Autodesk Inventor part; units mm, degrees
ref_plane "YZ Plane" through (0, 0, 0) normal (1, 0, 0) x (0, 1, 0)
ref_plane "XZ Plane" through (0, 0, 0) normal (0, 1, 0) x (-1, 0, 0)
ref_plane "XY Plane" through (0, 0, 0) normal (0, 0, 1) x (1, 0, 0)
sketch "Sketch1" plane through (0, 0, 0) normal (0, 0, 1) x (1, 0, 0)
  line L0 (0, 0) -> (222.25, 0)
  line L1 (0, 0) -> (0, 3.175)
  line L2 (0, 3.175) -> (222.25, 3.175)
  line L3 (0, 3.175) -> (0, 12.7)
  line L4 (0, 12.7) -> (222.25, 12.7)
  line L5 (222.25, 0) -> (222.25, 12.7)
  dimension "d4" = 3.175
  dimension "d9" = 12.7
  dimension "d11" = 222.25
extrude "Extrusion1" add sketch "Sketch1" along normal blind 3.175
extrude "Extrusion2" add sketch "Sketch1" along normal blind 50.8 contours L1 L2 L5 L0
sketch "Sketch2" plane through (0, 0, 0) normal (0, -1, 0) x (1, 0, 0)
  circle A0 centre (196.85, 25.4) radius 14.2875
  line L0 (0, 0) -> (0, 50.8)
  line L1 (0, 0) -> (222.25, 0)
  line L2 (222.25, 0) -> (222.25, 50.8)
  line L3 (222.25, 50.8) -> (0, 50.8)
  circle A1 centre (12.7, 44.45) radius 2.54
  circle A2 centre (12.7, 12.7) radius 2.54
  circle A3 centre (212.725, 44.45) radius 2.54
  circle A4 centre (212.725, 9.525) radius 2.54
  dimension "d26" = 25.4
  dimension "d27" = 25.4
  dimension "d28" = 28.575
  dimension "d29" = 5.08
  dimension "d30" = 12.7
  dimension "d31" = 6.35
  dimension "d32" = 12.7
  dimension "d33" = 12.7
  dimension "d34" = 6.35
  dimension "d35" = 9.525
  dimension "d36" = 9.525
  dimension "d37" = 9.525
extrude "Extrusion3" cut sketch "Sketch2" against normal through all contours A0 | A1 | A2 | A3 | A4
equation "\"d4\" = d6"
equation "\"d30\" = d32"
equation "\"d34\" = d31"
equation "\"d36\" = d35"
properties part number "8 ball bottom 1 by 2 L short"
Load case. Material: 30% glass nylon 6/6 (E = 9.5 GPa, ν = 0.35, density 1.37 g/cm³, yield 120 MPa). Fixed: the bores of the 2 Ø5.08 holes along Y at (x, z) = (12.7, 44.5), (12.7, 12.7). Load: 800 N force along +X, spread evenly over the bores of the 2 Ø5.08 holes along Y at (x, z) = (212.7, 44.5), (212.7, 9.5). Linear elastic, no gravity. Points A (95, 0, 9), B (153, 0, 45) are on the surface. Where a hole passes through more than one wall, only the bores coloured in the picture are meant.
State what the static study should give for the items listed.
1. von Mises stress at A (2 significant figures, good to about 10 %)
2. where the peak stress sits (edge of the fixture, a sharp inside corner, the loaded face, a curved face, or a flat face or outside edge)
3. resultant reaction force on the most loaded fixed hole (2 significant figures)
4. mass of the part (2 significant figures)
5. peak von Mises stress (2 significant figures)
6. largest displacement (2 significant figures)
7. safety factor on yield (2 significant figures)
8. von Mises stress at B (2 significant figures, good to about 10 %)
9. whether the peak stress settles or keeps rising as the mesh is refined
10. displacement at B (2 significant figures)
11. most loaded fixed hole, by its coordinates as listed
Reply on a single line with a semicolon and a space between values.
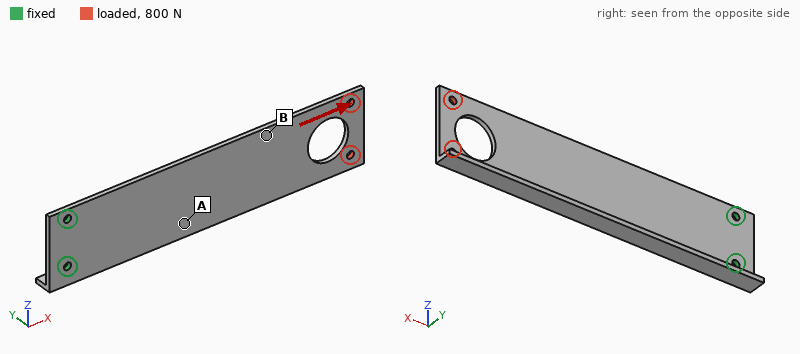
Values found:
4.6 MPa; a curved face; 440 N; 55 g; 26 MPa; 0.96 mm; 4.7; 7.5 MPa; settles; 0.40 mm; (12.7, 12.7)
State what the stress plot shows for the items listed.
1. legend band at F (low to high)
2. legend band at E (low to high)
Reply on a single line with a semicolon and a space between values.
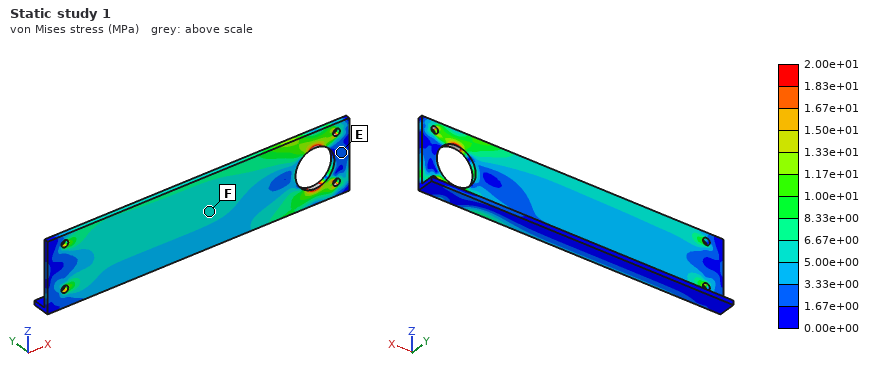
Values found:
5.00e+00 to 6.67e+00 MPa; 1.67e+00 to 3.33e+00 MPa
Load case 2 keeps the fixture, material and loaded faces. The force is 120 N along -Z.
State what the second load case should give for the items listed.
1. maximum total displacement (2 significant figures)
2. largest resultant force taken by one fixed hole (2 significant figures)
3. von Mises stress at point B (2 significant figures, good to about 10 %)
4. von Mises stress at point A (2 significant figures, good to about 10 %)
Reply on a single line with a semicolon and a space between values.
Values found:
2.5 mm; 710 N; 3.2 MPa; 7.2 MPa
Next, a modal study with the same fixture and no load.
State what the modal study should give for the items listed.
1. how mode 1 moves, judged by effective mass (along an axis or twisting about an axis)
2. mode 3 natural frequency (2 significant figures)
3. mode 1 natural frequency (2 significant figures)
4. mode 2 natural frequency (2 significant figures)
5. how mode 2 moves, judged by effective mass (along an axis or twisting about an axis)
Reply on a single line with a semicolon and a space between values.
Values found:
along Y; 370 Hz; 61 Hz; 230 Hz; twisting about X
